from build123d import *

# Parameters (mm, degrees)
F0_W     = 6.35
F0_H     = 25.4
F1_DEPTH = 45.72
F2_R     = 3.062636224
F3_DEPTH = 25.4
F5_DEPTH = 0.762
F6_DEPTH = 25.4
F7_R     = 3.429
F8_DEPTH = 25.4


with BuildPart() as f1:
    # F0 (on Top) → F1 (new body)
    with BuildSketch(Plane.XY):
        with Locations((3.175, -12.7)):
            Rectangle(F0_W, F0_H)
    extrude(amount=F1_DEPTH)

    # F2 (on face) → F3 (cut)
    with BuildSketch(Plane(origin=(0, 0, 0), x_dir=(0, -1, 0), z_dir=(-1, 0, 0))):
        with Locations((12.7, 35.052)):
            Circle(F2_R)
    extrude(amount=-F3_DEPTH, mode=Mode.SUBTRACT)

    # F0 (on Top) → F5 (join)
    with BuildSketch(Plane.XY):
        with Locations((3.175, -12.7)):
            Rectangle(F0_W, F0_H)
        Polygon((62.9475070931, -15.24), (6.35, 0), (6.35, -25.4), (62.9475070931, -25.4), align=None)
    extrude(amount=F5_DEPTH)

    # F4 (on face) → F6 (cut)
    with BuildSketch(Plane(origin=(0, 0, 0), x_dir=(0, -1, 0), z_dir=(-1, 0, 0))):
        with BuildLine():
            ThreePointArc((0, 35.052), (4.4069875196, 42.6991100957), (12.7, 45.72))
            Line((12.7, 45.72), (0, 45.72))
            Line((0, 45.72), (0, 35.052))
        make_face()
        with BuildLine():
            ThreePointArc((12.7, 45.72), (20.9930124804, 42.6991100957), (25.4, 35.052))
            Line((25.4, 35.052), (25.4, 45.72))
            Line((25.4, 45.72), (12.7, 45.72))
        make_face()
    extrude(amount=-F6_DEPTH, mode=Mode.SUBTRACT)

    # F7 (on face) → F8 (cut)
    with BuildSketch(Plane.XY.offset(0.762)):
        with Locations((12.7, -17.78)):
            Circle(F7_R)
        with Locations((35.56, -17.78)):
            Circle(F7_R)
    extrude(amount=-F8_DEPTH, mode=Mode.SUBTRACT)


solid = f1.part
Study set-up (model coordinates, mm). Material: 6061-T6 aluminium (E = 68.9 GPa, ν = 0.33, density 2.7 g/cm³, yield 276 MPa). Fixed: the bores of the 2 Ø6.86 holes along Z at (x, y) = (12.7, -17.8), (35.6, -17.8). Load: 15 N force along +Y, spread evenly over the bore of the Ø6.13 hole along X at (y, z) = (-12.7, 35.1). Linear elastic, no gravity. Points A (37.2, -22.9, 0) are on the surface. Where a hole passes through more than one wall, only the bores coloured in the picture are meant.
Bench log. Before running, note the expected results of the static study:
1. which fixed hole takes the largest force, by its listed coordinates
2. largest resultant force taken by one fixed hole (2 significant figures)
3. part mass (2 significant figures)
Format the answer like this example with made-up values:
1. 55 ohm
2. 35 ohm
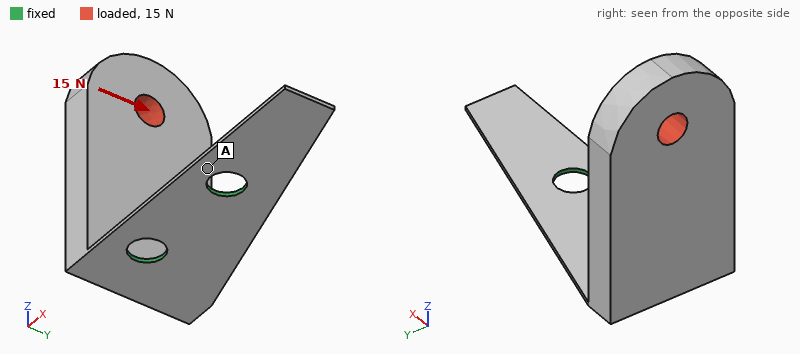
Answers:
1. (12.7, -17.8)
2. 16 N
3. 20 g
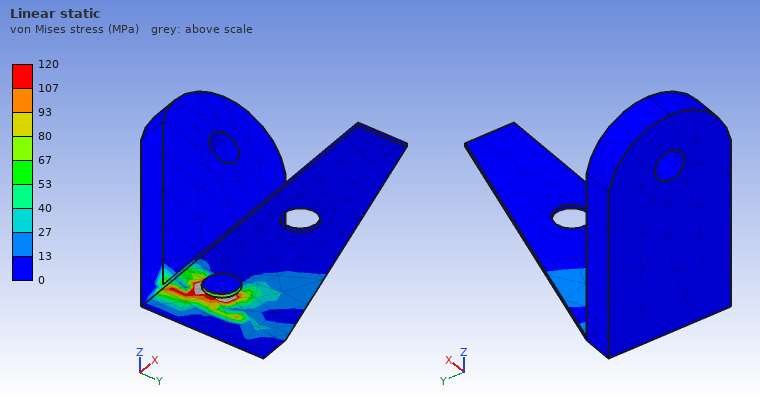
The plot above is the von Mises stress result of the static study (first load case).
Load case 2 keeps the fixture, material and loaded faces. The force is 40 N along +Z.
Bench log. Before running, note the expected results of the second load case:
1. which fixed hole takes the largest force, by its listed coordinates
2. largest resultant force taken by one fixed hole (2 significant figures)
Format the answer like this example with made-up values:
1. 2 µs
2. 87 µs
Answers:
1. (12.7, -17.8)
2. 41 N
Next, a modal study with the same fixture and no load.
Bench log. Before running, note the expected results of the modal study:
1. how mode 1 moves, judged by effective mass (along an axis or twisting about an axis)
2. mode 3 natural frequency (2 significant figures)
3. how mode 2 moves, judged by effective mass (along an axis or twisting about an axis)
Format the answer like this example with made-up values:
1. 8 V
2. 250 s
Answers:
1. along X
2. 1200 Hz
3. along Y
